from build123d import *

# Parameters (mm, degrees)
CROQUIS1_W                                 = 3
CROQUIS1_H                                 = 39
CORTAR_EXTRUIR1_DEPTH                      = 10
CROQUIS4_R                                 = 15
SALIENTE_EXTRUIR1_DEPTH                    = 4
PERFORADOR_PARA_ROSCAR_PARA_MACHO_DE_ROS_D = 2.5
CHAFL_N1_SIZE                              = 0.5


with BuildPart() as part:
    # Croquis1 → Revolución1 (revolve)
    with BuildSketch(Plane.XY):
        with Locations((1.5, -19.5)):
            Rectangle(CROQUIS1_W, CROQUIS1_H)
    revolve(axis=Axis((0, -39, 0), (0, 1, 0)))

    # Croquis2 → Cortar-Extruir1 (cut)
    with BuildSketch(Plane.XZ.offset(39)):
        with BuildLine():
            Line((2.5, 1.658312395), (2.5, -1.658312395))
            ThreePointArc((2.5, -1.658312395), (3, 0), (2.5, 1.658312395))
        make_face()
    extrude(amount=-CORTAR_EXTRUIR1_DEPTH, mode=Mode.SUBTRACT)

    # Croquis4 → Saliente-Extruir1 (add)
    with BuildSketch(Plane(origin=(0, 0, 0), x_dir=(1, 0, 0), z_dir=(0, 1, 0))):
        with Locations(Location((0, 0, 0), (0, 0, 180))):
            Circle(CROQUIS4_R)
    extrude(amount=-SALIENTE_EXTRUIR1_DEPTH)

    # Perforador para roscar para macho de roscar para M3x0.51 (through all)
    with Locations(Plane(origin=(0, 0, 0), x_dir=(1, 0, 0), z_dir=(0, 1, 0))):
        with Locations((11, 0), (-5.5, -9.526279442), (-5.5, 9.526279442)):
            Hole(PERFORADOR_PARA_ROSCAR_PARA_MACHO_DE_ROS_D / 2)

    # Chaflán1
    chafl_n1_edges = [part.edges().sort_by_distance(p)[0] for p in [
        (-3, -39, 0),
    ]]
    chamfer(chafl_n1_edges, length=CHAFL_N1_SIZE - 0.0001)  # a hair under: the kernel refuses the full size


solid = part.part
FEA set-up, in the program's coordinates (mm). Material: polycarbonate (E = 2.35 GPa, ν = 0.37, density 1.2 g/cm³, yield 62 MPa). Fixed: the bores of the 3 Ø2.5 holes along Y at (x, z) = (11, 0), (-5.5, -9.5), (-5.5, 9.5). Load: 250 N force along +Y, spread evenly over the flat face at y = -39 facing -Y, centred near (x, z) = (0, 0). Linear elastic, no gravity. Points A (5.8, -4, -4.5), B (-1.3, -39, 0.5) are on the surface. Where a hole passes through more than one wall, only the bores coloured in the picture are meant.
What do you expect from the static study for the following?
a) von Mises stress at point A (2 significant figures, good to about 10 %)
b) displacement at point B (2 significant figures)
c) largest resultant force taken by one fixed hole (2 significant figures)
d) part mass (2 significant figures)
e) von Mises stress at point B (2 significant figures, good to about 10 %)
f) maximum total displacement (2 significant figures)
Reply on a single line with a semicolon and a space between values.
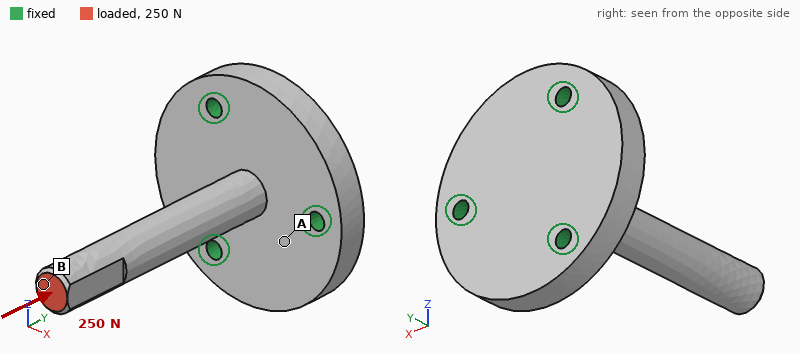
3.7 MPa; 0.19 mm; 84 N; 4.5 g; 8.0 MPa; 0.20 mm
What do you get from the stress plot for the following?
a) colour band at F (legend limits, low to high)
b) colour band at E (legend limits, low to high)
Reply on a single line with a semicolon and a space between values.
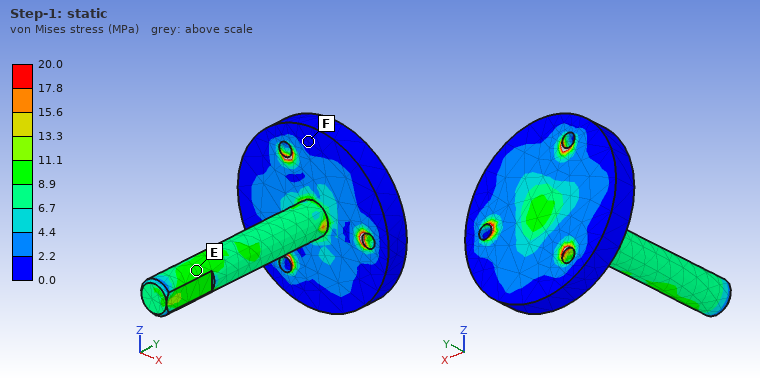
0.0 to 2.2 MPa; 8.9 to 11.1 MPa
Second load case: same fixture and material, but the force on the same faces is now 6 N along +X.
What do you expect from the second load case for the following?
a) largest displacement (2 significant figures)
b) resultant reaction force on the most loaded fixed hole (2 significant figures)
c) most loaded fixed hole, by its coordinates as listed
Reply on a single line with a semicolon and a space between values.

0.69 mm; 14 N; (11, 0)
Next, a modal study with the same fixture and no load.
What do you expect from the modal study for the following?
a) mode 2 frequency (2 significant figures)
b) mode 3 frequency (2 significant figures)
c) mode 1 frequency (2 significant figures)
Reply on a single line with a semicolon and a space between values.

870 Hz; 4900 Hz; 870 Hz
